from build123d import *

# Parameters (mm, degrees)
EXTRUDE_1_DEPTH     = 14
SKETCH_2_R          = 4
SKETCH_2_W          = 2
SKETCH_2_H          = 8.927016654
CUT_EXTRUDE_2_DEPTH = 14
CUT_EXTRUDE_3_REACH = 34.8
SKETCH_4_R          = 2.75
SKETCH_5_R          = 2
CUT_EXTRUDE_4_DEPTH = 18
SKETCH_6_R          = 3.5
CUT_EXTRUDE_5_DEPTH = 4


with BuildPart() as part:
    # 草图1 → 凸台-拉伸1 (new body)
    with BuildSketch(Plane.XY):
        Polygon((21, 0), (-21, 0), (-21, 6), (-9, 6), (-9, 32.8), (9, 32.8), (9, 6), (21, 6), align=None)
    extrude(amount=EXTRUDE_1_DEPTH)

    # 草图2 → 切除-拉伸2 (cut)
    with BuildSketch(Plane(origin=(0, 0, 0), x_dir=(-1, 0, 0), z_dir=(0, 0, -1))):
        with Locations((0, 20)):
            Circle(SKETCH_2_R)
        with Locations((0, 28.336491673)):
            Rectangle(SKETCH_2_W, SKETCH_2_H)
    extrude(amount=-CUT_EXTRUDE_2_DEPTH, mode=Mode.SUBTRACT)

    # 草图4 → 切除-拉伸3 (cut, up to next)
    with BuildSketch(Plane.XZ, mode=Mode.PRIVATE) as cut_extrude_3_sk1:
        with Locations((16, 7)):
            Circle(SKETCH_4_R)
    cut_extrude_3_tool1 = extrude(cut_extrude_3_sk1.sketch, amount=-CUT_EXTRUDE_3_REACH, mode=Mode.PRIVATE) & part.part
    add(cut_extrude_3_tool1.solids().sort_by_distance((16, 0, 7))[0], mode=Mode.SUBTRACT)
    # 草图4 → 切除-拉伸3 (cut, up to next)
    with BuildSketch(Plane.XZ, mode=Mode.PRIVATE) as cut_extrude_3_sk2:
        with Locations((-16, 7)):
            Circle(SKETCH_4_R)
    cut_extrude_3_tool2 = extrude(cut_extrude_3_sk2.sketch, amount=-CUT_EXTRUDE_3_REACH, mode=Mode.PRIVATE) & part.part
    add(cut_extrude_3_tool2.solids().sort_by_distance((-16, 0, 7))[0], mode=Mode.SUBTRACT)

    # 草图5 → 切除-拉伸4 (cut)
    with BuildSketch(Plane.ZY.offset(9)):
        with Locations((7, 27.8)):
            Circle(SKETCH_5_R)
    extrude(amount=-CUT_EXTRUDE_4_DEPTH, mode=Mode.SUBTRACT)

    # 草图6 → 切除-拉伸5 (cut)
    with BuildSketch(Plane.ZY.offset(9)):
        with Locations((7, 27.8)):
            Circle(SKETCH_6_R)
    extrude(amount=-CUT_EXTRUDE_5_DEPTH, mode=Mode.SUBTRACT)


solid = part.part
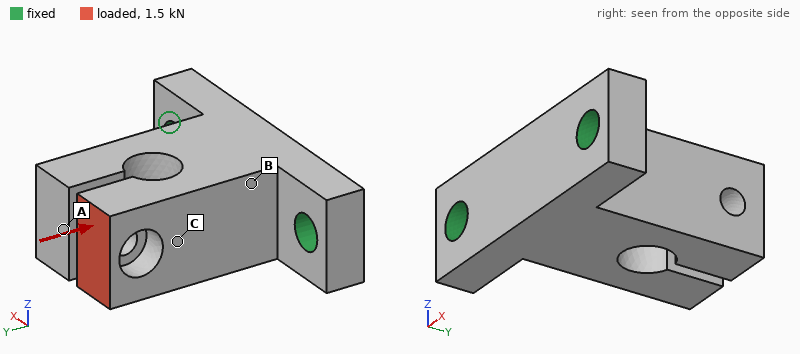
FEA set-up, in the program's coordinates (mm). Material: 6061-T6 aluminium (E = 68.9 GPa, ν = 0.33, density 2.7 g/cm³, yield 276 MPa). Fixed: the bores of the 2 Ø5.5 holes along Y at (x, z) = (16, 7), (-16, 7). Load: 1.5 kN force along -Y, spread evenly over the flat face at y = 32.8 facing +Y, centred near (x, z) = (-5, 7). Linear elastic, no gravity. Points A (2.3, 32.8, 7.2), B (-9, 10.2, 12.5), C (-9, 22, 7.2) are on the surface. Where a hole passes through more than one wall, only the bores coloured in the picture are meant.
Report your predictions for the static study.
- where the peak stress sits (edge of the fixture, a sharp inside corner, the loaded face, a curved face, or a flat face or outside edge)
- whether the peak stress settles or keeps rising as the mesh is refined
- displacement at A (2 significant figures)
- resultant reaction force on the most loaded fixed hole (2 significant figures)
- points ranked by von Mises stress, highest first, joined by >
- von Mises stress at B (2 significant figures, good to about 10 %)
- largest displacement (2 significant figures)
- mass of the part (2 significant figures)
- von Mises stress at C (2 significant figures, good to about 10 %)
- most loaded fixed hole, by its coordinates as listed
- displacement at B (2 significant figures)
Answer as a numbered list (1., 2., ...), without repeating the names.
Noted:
1. edge of the fixture
2. keeps rising
3. 9.1 µm
4. 1.1 kN
5. B > C > A
6. 19 MPa
7. 21 µm
8. 24 g
9. 12 MPa
10. (-16, 7)
11. 8.1 µm
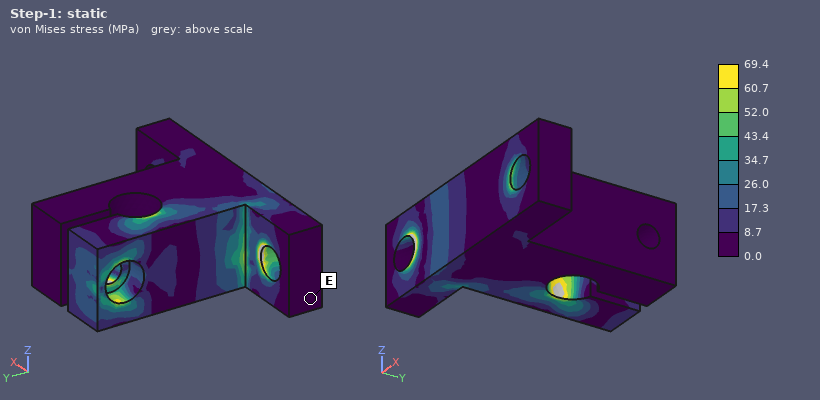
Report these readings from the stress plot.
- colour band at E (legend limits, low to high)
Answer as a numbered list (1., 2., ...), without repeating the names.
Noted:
1. 0.0 to 8.7 MPa
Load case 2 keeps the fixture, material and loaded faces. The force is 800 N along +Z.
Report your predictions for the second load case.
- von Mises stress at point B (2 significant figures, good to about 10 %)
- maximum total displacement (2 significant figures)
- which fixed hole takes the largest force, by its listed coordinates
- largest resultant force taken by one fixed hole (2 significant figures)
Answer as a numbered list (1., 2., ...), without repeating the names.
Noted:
1. 58 MPa
2. 0.18 mm
3. (-16, 7)
4. 520 N
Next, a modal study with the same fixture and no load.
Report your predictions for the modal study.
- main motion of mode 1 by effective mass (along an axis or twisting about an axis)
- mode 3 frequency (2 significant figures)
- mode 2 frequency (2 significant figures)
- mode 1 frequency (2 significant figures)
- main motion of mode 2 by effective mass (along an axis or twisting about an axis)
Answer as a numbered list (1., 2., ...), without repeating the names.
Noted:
1. along Z
2. 10 kHz
3. 8500 Hz
4. 5200 Hz
5. along X
